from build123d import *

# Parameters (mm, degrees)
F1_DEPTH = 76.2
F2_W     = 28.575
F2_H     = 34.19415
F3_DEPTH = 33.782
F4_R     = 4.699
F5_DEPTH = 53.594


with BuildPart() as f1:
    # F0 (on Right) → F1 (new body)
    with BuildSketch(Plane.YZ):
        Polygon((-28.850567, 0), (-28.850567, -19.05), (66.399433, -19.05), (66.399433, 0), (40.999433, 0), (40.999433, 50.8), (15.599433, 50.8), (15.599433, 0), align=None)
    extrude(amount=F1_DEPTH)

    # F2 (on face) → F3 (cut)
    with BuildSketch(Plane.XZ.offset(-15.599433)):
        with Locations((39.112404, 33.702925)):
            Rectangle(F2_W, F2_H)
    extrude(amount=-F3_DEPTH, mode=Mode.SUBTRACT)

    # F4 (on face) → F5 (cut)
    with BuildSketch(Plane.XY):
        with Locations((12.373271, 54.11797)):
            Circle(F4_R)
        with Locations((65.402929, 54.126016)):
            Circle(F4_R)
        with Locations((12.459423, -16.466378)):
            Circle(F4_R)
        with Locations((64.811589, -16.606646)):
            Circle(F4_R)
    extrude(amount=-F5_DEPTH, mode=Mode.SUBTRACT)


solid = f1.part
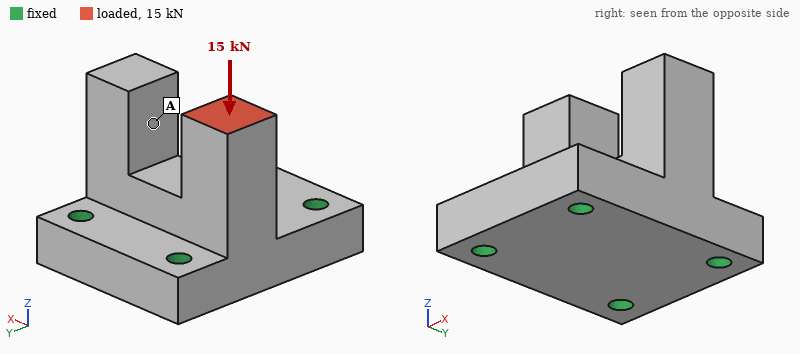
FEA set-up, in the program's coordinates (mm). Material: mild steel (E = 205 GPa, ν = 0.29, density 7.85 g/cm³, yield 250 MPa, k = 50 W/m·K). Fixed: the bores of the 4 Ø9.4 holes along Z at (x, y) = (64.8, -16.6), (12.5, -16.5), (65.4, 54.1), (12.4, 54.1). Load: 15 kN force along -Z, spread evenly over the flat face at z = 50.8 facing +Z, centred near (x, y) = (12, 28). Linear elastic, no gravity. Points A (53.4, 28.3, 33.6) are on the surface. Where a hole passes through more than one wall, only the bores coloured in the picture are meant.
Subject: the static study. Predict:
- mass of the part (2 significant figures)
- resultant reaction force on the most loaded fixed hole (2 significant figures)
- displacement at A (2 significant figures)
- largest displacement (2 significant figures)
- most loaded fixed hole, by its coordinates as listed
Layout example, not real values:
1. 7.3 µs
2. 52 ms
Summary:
1. 1.6 kg
2. 9.7 kN
3. 4.7 µm
4. 20 µm
5. (12.4, 54.1)
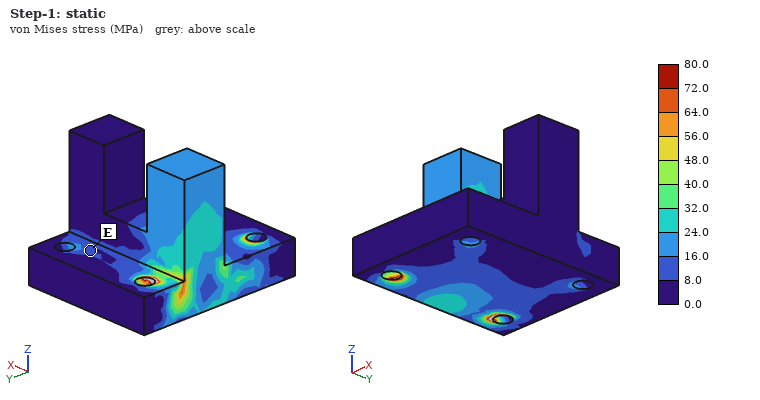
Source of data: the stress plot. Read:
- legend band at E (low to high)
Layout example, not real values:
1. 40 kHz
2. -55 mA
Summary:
1. 8.0 to 16.0 MPa
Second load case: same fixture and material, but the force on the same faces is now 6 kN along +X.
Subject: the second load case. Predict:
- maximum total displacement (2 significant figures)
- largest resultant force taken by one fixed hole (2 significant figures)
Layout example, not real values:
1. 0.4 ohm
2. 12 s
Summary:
1. 50 µm
2. 5.2 kN
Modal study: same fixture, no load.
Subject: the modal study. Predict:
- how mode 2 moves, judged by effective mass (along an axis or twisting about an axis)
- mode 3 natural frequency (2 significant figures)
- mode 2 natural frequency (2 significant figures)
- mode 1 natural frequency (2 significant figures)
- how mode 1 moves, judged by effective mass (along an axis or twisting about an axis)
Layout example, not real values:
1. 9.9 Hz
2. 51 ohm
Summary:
1. along X
2. 6400 Hz
3. 5700 Hz
4. 5400 Hz
5. along Y
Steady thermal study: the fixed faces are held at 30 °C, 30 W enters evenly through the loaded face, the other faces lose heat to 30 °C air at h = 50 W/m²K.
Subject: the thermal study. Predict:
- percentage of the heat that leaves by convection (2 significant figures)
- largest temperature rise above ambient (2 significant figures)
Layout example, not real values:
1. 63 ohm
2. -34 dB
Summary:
1. 29 %
2. 47 K
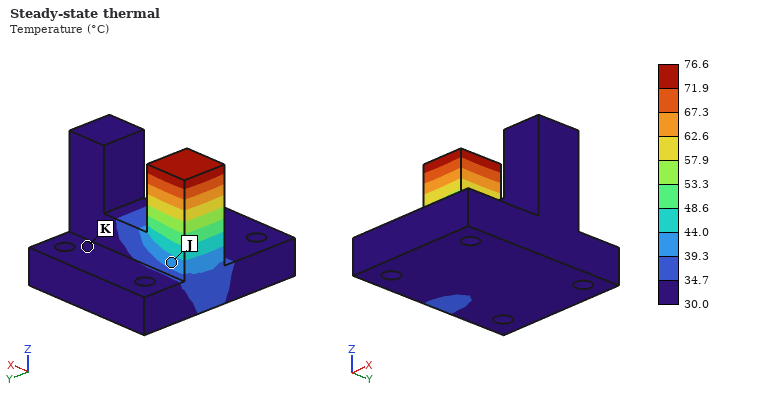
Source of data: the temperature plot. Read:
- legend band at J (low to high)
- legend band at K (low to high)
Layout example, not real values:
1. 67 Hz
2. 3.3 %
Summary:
1. 39.3 to 44.0 °C
2. 30.0 to 34.7 °C
